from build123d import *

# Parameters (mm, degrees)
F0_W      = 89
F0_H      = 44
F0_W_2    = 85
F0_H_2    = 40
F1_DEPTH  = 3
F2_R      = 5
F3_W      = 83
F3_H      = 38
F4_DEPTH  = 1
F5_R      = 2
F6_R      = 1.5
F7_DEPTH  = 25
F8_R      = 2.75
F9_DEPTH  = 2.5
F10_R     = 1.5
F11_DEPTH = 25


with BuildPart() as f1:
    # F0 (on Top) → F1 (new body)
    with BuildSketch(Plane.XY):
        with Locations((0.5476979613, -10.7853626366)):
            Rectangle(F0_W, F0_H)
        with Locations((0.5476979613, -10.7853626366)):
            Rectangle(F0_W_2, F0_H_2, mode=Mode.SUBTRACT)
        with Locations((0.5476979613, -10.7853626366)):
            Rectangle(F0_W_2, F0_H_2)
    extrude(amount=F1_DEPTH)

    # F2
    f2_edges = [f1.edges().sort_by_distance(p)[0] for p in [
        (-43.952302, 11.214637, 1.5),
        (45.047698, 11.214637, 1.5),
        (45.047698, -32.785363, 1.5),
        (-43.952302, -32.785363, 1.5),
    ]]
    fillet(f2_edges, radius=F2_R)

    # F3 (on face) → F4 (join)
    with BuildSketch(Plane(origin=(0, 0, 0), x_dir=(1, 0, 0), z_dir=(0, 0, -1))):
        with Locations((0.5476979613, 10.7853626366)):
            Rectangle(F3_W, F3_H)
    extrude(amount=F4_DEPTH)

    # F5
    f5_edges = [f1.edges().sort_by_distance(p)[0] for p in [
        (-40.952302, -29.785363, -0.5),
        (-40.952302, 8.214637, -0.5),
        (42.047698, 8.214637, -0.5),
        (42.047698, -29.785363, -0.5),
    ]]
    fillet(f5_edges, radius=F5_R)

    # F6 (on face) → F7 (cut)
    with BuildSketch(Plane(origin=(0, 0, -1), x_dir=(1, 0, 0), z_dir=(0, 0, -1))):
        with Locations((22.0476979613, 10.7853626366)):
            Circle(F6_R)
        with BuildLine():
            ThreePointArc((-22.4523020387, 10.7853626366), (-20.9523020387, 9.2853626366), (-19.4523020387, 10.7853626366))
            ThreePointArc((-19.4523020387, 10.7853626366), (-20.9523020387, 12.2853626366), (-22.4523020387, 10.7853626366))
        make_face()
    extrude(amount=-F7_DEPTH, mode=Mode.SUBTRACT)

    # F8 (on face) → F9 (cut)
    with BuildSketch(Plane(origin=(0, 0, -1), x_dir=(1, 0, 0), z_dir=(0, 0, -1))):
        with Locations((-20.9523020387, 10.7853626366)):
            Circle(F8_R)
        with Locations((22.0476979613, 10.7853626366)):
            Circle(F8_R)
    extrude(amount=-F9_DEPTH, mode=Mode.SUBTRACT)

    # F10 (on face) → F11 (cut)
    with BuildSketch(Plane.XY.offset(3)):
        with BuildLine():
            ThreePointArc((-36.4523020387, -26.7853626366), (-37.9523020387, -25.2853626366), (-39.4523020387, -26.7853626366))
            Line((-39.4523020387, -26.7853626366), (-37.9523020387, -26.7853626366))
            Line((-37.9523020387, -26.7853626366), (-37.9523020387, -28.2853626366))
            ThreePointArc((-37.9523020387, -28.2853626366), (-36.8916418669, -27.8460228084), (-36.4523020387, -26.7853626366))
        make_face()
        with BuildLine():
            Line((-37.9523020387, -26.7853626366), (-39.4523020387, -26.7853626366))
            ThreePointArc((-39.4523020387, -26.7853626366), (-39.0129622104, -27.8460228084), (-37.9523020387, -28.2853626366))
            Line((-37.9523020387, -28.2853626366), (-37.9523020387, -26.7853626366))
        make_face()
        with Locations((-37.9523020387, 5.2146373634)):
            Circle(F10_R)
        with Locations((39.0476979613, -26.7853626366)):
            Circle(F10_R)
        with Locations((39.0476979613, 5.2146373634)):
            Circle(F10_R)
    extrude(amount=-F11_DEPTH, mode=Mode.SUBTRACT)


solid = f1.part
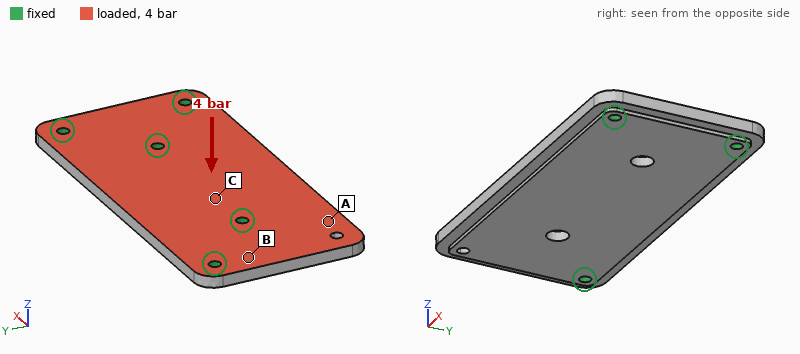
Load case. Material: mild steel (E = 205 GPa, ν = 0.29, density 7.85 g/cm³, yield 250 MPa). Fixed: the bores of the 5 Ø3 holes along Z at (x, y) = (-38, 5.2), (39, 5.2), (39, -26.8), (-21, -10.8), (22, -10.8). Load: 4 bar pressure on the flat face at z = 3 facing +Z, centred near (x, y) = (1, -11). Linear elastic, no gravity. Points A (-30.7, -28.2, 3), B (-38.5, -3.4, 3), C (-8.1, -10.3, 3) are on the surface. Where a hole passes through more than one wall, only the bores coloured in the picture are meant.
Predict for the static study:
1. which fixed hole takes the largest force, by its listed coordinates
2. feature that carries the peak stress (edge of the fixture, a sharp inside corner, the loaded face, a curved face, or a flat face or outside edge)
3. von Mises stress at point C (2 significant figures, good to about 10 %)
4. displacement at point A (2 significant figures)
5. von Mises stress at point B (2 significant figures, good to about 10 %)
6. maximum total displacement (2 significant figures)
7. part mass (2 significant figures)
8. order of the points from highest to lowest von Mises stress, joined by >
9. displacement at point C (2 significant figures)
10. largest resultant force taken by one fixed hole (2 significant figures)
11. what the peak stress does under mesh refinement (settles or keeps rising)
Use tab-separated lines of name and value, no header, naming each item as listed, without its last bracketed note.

which fixed hole takes the largest force, by its listed coordinates	(-21, -10.8)
feature that carries the peak stress	edge of the fixture
von Mises stress at point C	22 MPa
displacement at point A	19 µm
von Mises stress at point B	17 MPa
maximum total displacement	27 µm
part mass	110 g
order of the points from highest to lowest von Mises stress, joined by >	C > B > A
displacement at point C	6.3 µm
largest resultant force taken by one fixed hole	720 N
what the peak stress does under mesh refinement	keeps rising
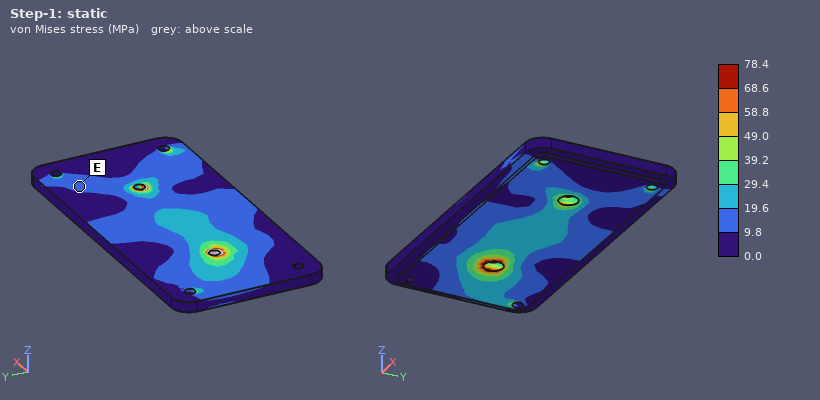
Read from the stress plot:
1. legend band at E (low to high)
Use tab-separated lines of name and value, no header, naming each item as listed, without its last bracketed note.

legend band at E	9.8 to 19.6 MPa
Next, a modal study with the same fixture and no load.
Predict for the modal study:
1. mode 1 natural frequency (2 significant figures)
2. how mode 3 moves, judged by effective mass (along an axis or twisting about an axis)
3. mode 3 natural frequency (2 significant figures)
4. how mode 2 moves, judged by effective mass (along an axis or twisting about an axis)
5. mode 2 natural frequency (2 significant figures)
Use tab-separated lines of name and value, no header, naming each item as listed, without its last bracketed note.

mode 1 natural frequency	4000 Hz
how mode 3 moves, judged by effective mass	along Z
mode 3 natural frequency	6200 Hz
how mode 2 moves, judged by effective mass	along Z
mode 2 natural frequency	5800 Hz
